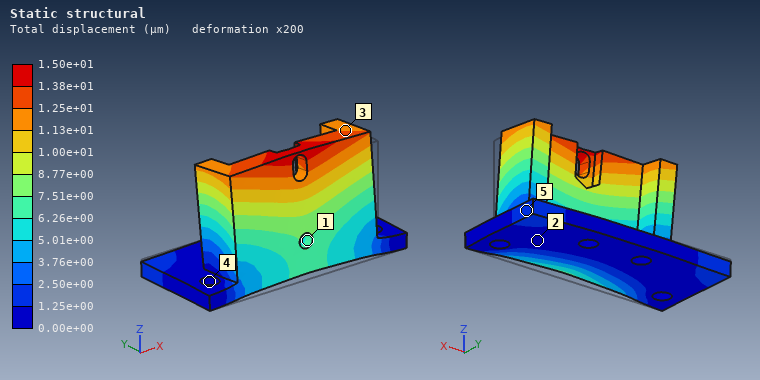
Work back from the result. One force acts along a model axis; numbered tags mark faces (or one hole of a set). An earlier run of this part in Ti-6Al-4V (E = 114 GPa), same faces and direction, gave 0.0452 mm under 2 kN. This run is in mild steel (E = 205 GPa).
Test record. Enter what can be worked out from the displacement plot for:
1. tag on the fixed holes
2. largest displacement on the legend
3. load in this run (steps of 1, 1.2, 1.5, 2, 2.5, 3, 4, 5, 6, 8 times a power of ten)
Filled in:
4
1.50e+01 µm
1.2 kN
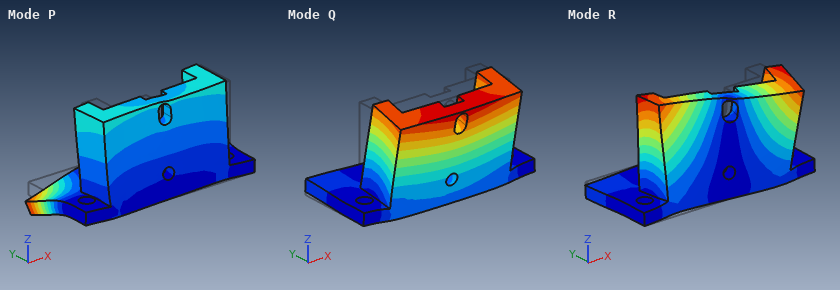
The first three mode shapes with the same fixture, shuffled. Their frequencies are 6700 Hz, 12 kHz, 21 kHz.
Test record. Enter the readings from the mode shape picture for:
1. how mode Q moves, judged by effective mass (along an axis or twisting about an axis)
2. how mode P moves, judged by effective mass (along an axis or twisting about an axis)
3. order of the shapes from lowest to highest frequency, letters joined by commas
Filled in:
along Y
along X
Q, R, P
